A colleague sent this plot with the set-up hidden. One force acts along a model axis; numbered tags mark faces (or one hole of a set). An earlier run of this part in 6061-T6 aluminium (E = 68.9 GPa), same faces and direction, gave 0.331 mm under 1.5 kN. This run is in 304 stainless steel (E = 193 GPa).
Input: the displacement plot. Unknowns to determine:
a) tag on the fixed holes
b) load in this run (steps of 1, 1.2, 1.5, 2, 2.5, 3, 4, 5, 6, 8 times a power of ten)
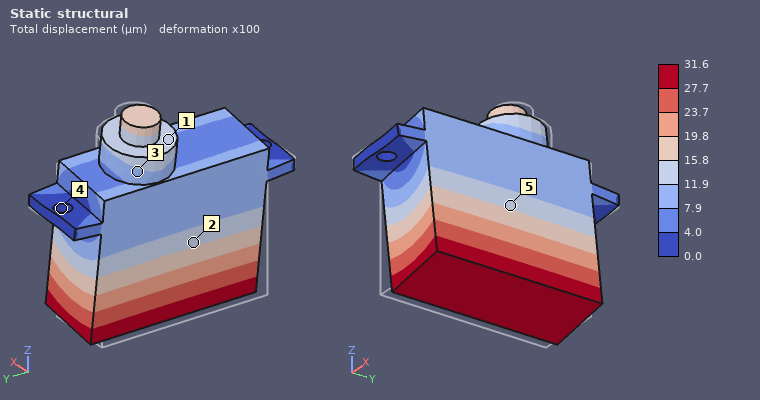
4
400 N
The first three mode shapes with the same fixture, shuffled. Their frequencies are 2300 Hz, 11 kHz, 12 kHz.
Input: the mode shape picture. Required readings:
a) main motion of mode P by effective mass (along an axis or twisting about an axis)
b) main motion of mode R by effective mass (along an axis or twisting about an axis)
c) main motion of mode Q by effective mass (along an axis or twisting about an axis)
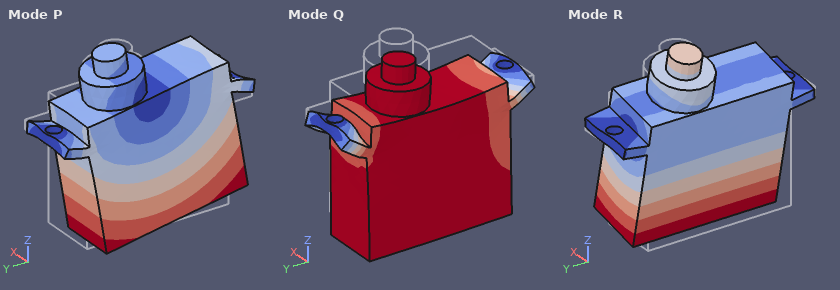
along Y
along X
along Z
